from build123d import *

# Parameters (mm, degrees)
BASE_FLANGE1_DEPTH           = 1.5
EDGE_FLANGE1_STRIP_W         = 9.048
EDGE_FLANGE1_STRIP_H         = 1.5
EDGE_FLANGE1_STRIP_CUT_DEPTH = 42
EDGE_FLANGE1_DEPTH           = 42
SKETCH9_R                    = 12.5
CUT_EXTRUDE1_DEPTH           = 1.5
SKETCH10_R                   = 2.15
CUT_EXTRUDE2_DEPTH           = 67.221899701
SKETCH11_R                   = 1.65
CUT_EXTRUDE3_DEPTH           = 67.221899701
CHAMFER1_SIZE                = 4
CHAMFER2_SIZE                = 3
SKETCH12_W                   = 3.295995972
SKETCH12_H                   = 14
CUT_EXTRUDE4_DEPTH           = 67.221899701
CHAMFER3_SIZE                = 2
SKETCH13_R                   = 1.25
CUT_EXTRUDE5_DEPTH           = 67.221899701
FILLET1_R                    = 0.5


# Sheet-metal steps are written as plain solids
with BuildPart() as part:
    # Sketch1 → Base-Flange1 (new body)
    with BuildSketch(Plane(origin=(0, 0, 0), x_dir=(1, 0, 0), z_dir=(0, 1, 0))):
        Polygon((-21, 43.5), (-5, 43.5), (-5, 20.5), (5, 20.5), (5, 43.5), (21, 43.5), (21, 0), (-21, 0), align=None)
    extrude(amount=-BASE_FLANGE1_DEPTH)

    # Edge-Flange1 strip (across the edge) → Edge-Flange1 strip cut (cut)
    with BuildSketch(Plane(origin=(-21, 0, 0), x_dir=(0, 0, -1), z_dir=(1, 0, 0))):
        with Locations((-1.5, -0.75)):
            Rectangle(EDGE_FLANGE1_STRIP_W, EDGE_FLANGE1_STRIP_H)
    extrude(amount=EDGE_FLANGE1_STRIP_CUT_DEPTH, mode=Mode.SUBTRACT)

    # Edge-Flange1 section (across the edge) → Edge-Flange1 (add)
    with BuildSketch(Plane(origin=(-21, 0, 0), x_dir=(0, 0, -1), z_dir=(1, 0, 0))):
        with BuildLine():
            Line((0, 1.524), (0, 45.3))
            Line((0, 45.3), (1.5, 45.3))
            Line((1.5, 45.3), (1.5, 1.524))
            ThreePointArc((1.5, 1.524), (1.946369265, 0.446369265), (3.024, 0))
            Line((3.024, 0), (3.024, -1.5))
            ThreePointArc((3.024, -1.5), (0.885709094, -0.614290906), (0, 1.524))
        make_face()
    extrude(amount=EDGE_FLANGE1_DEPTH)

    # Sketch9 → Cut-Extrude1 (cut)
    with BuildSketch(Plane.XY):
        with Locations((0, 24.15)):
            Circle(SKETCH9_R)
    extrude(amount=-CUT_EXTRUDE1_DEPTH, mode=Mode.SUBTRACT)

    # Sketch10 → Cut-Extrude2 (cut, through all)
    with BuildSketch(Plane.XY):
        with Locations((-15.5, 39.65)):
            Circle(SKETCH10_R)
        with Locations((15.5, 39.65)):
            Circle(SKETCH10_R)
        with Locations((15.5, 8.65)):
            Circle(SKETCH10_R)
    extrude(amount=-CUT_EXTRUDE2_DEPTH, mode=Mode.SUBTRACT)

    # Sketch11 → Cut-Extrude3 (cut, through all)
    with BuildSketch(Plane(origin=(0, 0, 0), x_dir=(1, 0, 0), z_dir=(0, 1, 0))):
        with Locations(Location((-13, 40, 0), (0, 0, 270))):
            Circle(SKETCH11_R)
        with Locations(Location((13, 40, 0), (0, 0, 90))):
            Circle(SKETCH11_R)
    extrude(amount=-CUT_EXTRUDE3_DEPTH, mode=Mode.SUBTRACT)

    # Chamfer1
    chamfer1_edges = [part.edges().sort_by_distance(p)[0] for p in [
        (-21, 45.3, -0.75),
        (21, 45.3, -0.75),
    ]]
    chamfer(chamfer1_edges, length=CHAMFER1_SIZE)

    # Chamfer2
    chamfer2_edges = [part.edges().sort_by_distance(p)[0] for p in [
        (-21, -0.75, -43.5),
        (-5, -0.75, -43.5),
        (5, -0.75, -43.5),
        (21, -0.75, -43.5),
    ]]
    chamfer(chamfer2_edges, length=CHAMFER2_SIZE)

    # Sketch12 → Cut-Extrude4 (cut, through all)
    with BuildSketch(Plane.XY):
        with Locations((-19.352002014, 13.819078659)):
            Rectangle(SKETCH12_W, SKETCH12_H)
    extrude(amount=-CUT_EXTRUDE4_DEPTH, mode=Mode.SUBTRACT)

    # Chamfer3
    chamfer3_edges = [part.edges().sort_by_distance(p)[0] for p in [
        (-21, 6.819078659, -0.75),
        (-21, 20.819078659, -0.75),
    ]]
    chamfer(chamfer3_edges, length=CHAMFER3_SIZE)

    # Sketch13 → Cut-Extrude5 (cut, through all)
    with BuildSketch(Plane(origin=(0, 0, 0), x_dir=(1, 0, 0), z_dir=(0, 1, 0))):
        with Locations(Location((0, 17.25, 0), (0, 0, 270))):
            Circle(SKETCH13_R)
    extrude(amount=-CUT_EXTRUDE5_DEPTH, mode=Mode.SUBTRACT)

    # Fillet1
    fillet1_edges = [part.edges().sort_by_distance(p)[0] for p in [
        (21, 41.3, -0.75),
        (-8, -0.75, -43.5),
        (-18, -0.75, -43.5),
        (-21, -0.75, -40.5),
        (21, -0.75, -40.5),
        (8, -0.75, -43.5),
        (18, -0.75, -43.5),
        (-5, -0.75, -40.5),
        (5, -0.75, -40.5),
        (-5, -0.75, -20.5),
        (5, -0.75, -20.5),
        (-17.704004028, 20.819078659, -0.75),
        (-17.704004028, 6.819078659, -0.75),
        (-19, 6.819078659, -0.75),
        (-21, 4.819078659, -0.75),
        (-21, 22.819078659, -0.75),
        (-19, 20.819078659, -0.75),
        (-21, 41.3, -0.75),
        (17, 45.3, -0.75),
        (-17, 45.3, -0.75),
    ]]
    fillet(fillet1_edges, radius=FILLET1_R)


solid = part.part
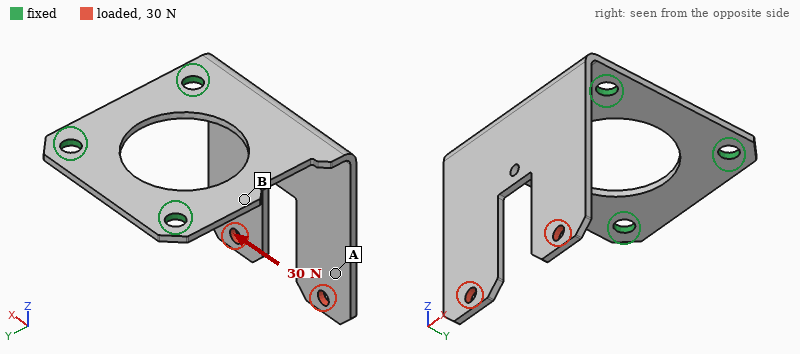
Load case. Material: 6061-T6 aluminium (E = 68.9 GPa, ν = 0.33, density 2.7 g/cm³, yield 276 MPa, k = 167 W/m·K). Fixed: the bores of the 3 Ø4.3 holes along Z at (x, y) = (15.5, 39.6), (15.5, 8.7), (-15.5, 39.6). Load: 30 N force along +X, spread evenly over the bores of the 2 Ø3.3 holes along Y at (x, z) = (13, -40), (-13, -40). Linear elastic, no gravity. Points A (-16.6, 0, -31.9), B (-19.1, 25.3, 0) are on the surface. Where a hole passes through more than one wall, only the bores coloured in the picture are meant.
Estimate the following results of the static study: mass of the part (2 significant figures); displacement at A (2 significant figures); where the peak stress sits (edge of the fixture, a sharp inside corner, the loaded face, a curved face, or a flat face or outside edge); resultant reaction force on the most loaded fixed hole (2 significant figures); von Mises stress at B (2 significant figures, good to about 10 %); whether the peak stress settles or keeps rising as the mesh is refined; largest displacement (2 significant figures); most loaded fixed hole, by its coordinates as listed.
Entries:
11 g
0.58 mm
edge of the fixture
31 N
28 MPa
keeps rising
0.73 mm
(15.5, 8.7)
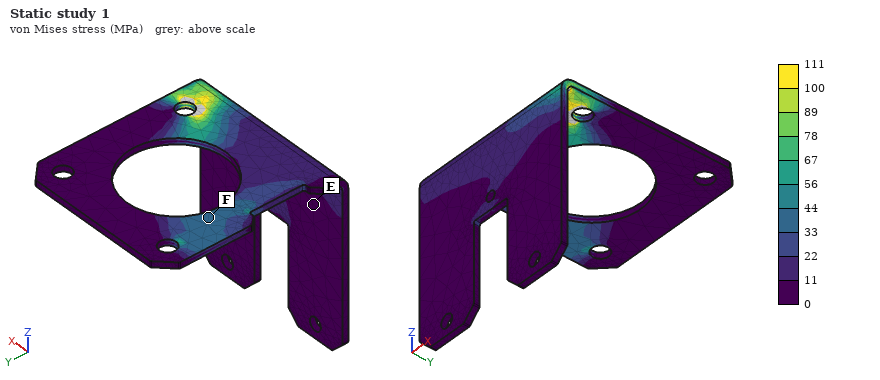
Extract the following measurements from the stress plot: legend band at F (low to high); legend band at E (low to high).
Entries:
33 to 44 MPa
0 to 11 MPa
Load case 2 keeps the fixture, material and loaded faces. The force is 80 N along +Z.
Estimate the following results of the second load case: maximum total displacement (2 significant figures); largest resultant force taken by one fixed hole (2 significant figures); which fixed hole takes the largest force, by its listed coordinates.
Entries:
0.90 mm
78 N
(15.5, 8.7)
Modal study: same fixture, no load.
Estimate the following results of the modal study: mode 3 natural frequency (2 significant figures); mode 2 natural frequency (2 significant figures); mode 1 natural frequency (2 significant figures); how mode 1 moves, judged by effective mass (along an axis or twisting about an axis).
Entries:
1000 Hz
760 Hz
480 Hz
along Y
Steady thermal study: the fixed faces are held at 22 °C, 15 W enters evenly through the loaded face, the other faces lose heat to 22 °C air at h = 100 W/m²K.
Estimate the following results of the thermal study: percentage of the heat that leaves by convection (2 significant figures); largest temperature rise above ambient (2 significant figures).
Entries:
68 %
59 K
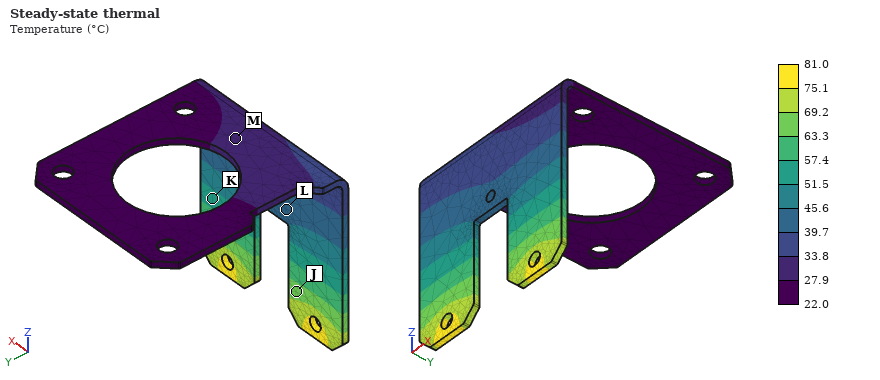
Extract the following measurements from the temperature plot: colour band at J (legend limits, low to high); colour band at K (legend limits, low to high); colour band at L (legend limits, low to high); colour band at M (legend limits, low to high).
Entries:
63.3 to 69.2 °C
51.5 to 57.4 °C
39.7 to 45.6 °C
27.9 to 33.8 °C
